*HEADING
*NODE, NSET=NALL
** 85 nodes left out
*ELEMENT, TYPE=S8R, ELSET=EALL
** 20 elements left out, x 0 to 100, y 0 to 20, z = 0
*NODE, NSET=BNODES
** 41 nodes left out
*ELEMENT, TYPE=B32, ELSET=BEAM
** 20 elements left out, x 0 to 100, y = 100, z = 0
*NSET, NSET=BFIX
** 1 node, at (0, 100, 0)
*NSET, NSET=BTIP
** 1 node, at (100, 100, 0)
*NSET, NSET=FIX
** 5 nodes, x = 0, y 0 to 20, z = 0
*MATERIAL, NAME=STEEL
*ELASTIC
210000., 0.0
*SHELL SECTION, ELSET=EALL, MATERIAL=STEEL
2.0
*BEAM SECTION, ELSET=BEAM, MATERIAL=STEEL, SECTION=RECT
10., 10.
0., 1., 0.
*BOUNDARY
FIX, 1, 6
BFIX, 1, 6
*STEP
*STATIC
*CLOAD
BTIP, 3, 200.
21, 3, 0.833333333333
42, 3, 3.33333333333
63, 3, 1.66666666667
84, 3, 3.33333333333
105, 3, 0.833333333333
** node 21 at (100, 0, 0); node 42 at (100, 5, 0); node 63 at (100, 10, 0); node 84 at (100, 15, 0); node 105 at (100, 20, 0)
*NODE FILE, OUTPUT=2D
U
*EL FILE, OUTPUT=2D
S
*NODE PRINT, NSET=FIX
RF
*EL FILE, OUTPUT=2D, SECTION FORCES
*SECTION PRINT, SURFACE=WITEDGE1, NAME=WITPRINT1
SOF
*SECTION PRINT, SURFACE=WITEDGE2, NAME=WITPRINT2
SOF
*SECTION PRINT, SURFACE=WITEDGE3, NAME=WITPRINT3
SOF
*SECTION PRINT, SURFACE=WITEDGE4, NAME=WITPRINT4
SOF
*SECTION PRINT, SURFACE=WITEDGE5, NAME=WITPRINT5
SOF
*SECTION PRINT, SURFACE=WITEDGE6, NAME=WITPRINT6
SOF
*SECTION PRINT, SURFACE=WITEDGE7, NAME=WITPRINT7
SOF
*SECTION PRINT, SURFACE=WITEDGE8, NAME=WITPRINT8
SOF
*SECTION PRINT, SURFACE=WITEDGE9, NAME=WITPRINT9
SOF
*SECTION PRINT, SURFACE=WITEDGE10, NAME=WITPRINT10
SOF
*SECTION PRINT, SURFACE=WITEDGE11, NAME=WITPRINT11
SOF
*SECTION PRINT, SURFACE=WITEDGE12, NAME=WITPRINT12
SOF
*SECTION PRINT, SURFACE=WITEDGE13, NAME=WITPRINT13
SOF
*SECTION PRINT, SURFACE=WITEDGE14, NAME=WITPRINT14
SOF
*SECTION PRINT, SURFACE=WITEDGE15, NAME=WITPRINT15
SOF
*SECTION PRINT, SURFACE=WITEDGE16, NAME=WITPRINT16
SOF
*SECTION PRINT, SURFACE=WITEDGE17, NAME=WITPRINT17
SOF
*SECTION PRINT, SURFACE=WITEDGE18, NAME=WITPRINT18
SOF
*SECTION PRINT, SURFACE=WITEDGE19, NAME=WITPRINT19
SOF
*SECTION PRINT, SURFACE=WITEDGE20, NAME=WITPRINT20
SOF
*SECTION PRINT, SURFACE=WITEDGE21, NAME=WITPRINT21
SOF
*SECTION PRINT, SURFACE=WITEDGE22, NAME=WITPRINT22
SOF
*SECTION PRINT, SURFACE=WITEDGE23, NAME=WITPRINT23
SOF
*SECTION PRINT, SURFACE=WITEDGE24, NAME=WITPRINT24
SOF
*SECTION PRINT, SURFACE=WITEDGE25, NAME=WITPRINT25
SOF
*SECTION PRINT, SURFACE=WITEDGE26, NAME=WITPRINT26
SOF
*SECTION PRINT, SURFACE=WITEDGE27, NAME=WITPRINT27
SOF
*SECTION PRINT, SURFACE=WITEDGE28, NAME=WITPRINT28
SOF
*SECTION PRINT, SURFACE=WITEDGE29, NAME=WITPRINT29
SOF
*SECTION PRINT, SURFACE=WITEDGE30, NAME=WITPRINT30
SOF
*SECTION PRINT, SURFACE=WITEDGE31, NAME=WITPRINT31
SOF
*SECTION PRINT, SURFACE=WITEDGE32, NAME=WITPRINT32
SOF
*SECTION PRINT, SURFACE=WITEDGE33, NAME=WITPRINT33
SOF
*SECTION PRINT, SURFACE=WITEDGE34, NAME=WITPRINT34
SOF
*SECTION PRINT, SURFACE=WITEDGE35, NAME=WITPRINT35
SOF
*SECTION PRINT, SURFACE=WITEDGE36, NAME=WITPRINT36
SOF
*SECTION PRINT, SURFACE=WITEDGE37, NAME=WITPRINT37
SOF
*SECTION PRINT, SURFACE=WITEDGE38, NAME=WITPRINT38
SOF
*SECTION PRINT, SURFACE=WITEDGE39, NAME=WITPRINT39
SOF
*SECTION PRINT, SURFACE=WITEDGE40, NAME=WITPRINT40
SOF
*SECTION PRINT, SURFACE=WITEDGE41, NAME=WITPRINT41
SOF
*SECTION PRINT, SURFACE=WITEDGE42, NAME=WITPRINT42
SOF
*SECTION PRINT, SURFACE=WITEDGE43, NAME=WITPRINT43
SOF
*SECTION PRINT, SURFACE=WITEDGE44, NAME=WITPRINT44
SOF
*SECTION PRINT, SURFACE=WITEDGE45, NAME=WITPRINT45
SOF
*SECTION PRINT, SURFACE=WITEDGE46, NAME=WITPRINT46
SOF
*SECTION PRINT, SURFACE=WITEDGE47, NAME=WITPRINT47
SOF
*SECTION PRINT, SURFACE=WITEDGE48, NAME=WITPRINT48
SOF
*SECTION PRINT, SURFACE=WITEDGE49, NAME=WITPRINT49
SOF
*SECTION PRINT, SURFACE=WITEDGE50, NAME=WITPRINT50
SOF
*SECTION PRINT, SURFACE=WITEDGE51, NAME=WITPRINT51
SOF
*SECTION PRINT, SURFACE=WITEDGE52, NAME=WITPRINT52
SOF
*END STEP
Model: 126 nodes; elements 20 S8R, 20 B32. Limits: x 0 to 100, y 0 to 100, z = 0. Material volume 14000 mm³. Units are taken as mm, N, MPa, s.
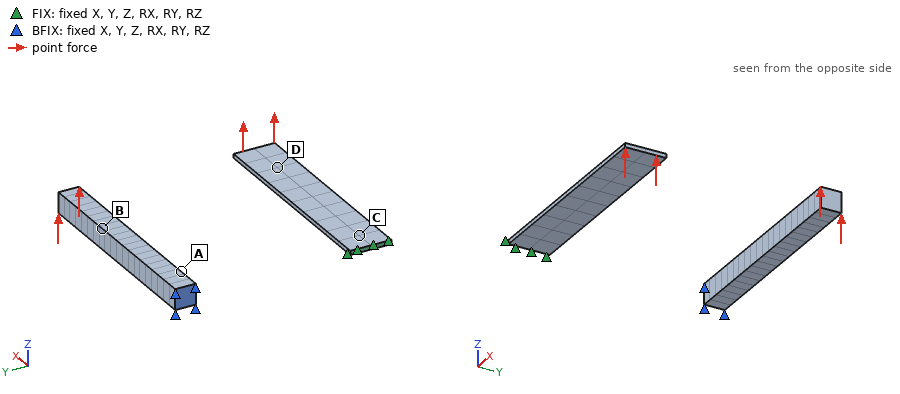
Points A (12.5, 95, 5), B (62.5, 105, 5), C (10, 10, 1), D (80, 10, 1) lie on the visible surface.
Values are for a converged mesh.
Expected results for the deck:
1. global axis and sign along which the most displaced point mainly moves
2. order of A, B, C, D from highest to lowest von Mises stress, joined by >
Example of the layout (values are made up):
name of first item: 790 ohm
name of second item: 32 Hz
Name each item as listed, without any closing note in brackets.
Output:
global axis and sign along which the most displaced point mainly moves: +Z
order of A, B, C, D from highest to lowest von Mises stress, joined by >: A > C > B > D
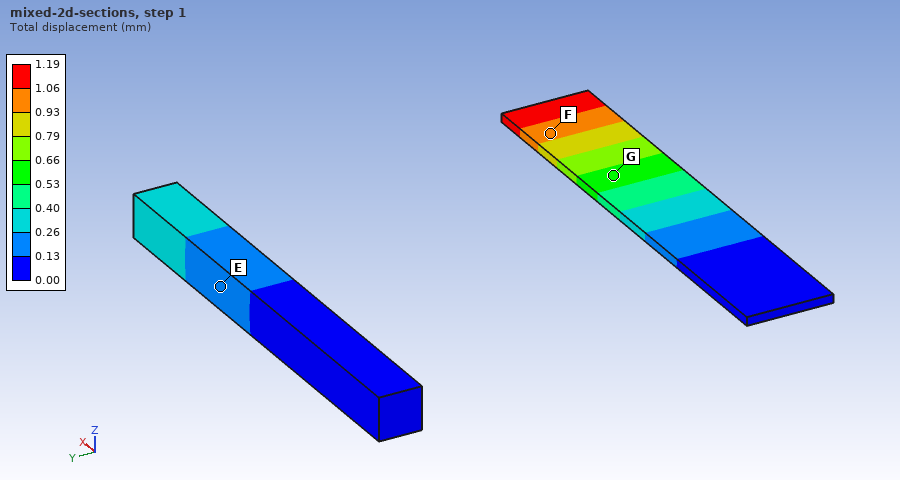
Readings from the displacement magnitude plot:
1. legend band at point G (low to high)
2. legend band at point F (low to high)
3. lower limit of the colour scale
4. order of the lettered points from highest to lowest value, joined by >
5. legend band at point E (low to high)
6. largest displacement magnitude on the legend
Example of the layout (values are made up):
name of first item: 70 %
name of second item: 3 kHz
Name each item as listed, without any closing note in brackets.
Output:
legend band at point G: 0.53 to 0.66 mm
legend band at point F: 0.93 to 1.06 mm
lower limit of the colour scale: 0.00 mm
order of the lettered points from highest to lowest value, joined by >: F > G > E
legend band at point E: 0.13 to 0.26 mm
largest displacement magnitude on the legend: 1.19 mm
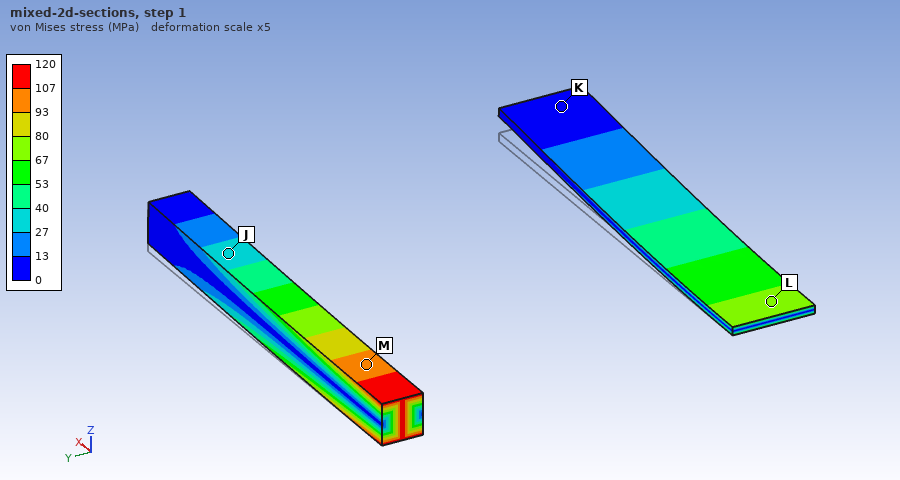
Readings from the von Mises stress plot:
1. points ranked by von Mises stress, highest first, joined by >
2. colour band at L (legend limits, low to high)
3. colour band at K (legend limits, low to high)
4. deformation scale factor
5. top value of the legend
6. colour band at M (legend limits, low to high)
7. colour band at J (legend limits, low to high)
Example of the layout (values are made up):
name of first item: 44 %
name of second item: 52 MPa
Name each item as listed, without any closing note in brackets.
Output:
points ranked by von Mises stress, highest first, joined by >: M > L > J > K
colour band at L: 67 to 80 MPa
colour band at K: 0 to 13 MPa
deformation scale factor: 5
top value of the legend: 120 MPa
colour band at M: 93 to 107 MPa
colour band at J: 27 to 40 MPa
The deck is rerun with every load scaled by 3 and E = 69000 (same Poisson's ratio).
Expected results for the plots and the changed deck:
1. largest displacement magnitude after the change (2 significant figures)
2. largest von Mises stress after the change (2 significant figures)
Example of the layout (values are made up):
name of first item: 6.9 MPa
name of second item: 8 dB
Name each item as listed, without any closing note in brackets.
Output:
largest displacement magnitude after the change: 11 mm
largest von Mises stress after the change: 360 MPa
